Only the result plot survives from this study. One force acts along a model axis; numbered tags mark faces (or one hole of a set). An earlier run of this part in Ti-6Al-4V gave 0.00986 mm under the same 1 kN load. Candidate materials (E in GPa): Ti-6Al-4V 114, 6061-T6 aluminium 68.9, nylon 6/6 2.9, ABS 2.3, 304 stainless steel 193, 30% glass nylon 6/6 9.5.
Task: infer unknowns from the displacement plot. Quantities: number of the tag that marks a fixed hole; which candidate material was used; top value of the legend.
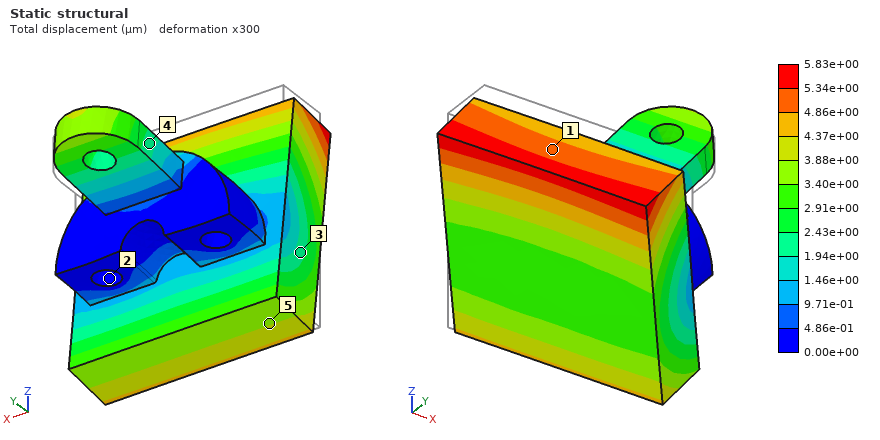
2
304 stainless steel
5.83e+00 µm
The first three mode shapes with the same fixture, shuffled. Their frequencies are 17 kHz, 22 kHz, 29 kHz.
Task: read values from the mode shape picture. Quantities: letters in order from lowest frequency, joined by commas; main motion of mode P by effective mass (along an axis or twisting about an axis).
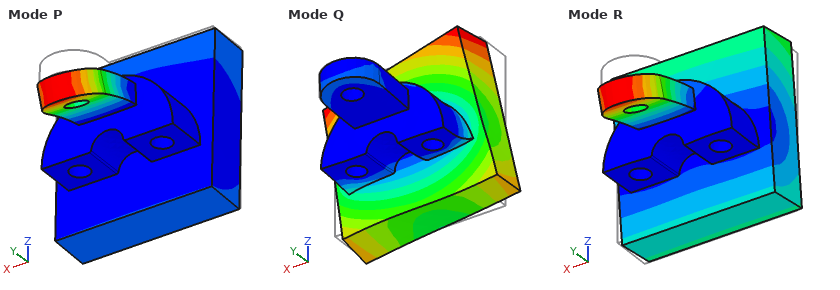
R, P, Q
along Z
